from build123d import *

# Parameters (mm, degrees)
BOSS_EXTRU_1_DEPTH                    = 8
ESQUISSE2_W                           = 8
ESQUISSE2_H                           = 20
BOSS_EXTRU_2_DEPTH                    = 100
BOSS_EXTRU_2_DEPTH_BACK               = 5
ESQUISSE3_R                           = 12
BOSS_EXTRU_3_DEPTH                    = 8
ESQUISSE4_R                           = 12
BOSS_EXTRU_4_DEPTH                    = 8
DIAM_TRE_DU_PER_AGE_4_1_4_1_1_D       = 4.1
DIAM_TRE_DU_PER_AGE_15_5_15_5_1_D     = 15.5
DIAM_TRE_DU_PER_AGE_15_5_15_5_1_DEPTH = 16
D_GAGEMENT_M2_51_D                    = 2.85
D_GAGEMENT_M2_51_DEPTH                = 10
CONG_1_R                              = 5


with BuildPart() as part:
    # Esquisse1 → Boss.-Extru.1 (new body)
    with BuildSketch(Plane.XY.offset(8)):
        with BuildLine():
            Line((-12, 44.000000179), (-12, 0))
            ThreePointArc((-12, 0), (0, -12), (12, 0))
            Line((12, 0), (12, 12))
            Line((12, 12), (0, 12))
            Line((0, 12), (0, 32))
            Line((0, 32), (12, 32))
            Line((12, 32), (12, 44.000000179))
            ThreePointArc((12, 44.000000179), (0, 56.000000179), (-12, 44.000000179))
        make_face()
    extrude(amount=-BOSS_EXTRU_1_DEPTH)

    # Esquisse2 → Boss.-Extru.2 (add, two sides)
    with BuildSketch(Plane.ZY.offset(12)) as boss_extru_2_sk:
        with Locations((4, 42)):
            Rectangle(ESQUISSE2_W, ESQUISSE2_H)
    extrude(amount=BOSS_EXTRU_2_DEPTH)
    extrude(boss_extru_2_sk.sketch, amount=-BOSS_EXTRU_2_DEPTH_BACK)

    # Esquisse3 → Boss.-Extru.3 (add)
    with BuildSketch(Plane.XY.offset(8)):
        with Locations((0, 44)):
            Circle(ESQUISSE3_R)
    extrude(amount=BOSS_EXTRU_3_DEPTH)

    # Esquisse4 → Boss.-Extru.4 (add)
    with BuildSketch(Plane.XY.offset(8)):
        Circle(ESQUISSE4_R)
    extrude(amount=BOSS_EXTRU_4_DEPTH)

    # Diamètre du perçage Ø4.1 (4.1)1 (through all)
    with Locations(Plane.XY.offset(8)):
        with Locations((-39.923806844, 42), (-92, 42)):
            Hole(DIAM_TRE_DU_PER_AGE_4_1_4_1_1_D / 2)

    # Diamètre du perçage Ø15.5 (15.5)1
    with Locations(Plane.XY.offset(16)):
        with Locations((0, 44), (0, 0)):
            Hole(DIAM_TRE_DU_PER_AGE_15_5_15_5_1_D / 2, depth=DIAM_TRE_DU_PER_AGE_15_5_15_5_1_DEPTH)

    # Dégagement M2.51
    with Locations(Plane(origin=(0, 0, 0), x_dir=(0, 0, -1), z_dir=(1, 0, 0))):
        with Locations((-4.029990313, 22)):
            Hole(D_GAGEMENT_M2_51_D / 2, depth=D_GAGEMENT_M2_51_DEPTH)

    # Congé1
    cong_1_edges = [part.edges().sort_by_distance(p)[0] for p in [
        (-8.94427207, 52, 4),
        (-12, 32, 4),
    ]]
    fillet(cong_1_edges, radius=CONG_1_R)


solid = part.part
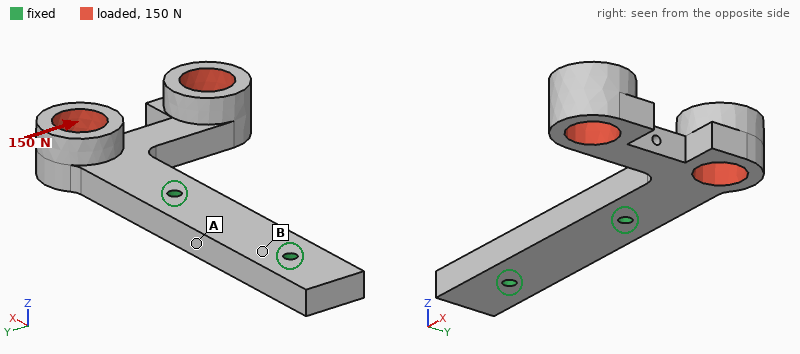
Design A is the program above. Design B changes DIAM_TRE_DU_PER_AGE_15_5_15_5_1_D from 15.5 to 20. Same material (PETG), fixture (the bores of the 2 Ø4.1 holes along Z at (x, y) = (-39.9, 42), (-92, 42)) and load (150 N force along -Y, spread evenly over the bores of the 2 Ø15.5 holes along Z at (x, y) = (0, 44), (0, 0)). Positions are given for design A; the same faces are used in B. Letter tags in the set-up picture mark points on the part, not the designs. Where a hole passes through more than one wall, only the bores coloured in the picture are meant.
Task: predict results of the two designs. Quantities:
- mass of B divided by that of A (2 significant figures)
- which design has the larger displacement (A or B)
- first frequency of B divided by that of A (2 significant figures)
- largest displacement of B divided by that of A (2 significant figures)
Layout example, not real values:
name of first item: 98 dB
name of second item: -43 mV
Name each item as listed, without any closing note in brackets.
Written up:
mass of B divided by that of A: 0.85
which design has the larger displacement: B
first frequency of B divided by that of A: 1.2
largest displacement of B divided by that of A: 1.4
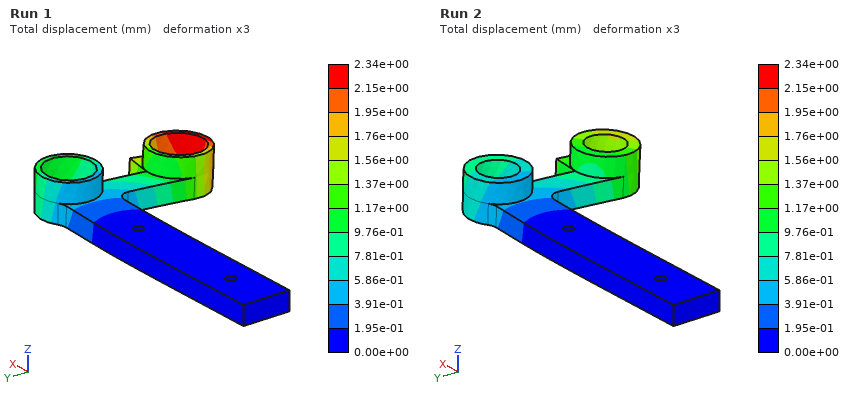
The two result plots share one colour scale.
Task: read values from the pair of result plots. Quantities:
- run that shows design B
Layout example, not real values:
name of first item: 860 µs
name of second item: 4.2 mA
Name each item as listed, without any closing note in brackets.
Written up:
run that shows design B: Run 1
